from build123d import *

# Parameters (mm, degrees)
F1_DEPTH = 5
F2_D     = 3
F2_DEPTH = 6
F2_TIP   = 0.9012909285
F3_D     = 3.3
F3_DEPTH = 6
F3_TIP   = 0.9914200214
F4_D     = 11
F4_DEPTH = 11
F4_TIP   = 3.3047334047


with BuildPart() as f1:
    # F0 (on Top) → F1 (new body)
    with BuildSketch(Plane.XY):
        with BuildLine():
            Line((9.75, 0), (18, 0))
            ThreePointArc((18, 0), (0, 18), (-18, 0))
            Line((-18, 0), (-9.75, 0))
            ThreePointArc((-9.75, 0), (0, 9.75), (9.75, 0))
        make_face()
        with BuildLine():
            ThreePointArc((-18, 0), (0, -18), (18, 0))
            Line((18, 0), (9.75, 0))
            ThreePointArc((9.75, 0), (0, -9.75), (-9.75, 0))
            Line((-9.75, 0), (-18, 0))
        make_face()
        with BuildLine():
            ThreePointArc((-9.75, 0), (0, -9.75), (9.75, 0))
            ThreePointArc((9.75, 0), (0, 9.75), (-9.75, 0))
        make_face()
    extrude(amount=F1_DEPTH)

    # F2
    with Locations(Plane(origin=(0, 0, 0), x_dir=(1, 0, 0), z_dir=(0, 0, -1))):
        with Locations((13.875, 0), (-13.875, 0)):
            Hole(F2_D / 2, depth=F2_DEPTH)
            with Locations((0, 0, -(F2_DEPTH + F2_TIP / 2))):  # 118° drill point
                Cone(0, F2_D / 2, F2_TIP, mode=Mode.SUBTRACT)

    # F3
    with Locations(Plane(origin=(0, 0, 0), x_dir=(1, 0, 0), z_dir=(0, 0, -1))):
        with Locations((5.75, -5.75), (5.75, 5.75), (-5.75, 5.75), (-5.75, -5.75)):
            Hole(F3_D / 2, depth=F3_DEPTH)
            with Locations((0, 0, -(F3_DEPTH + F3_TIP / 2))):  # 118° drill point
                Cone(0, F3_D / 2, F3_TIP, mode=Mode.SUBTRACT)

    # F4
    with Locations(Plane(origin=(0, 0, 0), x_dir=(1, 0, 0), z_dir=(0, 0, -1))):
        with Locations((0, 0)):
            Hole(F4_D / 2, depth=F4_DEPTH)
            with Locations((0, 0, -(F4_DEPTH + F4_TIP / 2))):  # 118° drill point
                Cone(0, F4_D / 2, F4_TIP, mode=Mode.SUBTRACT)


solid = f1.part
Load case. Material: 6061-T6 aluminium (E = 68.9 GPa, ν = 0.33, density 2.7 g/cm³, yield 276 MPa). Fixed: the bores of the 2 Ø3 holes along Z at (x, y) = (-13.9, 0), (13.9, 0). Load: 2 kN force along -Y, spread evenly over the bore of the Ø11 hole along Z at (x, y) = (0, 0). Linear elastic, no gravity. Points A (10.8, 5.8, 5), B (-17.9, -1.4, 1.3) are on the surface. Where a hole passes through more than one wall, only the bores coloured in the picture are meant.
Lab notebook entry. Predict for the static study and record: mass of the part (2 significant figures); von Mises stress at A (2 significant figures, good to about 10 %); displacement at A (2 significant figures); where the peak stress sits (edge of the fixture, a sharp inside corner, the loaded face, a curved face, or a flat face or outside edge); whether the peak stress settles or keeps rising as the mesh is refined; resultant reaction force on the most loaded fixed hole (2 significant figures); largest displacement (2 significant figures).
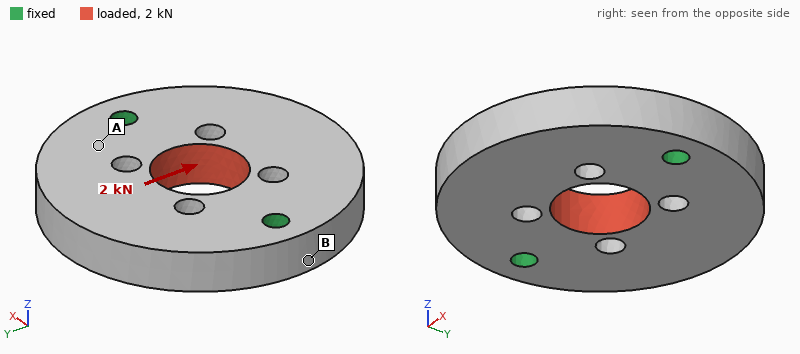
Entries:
12 g
18 MPa
2.0 µm
edge of the fixture
keeps rising
1.0 kN
5.5 µm
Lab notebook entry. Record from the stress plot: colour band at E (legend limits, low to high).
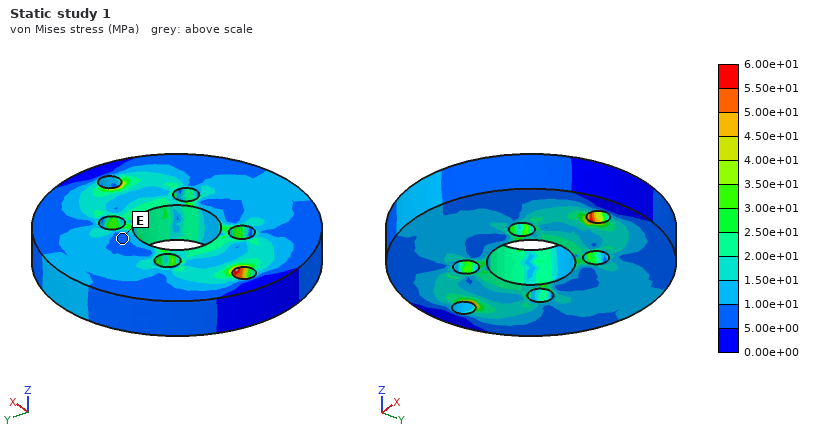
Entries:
5.00e+00 to 1.00e+01 MPa
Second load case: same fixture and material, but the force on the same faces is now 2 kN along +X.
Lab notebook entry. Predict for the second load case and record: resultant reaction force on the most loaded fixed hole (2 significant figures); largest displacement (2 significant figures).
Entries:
1.0 kN
4.7 µm
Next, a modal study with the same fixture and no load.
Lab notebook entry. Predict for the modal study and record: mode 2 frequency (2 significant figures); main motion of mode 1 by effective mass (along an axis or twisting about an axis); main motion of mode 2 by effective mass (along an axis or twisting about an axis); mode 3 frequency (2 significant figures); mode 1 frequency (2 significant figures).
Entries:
12 kHz
twisting about X
along Z
27 kHz
10 kHz
